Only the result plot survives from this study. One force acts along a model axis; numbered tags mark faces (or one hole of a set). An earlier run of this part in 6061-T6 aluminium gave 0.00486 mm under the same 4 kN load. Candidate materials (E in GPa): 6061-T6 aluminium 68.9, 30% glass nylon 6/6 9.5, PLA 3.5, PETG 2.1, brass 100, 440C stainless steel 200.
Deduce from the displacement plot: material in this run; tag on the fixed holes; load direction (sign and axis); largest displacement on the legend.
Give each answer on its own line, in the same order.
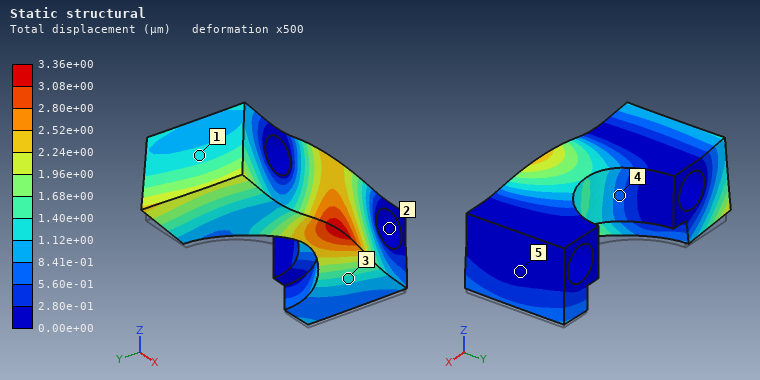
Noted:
brass
2
+Z
3.36e+00 µm
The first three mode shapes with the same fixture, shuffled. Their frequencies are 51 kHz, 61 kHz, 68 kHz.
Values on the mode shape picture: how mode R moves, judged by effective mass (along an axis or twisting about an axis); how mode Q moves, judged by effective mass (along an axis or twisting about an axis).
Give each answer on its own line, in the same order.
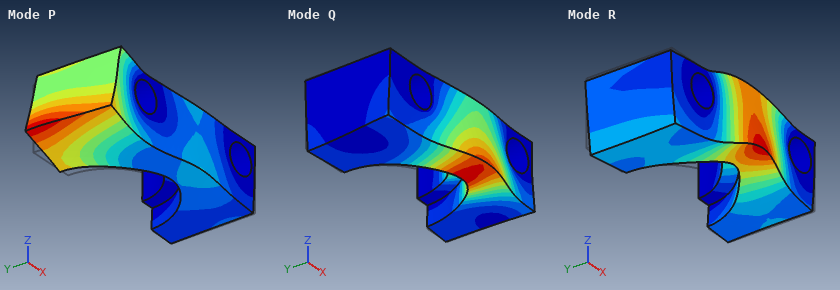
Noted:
along Z
along Y
